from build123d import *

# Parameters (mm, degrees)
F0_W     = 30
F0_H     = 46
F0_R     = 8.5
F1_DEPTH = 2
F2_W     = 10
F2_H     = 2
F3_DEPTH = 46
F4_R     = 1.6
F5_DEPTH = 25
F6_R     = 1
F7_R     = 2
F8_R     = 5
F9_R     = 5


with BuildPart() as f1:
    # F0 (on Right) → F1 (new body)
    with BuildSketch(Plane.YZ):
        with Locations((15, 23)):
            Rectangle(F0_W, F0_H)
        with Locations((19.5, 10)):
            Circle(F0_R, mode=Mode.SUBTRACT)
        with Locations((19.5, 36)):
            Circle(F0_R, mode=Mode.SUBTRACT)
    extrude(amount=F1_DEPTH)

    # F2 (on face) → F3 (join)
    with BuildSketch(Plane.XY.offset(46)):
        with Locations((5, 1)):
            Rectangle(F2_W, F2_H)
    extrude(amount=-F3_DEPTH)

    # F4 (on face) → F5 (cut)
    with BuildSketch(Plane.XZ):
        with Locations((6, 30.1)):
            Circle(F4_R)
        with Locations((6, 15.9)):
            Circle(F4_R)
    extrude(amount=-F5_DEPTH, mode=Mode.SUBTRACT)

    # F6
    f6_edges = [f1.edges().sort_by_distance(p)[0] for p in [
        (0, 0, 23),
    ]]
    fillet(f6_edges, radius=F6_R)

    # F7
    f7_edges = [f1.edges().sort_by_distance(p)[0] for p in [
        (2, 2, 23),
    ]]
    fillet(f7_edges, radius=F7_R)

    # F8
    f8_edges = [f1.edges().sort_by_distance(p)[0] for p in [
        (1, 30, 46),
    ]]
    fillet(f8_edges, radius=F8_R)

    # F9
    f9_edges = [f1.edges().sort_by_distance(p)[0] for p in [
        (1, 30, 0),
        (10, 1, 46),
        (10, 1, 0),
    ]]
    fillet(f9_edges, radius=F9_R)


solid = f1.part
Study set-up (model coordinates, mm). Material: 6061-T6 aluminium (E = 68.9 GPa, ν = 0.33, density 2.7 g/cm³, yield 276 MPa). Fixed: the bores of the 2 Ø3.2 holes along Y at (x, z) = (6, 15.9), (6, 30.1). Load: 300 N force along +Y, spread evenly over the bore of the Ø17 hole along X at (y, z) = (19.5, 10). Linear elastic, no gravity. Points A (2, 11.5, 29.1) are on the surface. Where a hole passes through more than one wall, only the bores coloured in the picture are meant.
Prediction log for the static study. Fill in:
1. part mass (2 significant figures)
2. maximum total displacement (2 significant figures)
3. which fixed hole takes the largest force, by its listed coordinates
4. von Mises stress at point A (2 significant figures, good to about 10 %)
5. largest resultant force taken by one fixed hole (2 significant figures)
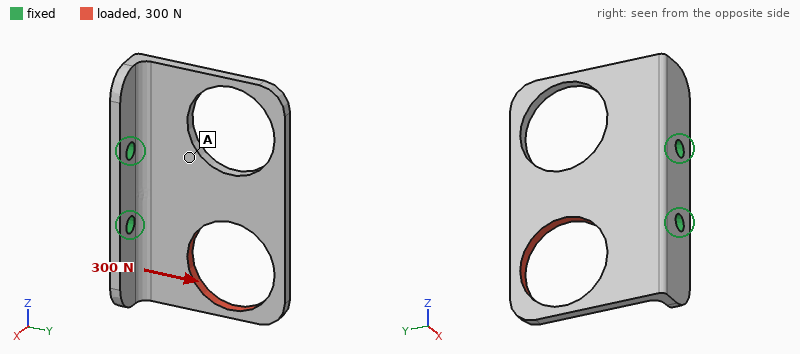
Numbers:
6.9 g
0.12 mm
(6, 15.9)
17 MPa
380 N
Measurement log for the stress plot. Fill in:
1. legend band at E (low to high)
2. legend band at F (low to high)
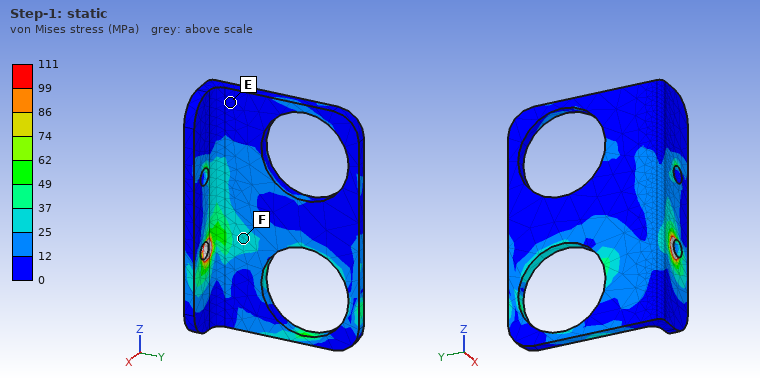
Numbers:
0 to 12 MPa
25 to 37 MPa
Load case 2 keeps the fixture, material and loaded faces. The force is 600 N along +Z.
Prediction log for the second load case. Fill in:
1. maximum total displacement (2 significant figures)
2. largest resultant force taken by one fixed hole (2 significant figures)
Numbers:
0.20 mm
750 N
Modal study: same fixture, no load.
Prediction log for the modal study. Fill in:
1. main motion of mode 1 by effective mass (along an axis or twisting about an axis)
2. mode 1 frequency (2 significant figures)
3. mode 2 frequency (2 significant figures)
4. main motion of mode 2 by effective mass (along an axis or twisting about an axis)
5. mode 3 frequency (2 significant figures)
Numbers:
along X
1900 Hz
3300 Hz
twisting about Y
6100 Hz
